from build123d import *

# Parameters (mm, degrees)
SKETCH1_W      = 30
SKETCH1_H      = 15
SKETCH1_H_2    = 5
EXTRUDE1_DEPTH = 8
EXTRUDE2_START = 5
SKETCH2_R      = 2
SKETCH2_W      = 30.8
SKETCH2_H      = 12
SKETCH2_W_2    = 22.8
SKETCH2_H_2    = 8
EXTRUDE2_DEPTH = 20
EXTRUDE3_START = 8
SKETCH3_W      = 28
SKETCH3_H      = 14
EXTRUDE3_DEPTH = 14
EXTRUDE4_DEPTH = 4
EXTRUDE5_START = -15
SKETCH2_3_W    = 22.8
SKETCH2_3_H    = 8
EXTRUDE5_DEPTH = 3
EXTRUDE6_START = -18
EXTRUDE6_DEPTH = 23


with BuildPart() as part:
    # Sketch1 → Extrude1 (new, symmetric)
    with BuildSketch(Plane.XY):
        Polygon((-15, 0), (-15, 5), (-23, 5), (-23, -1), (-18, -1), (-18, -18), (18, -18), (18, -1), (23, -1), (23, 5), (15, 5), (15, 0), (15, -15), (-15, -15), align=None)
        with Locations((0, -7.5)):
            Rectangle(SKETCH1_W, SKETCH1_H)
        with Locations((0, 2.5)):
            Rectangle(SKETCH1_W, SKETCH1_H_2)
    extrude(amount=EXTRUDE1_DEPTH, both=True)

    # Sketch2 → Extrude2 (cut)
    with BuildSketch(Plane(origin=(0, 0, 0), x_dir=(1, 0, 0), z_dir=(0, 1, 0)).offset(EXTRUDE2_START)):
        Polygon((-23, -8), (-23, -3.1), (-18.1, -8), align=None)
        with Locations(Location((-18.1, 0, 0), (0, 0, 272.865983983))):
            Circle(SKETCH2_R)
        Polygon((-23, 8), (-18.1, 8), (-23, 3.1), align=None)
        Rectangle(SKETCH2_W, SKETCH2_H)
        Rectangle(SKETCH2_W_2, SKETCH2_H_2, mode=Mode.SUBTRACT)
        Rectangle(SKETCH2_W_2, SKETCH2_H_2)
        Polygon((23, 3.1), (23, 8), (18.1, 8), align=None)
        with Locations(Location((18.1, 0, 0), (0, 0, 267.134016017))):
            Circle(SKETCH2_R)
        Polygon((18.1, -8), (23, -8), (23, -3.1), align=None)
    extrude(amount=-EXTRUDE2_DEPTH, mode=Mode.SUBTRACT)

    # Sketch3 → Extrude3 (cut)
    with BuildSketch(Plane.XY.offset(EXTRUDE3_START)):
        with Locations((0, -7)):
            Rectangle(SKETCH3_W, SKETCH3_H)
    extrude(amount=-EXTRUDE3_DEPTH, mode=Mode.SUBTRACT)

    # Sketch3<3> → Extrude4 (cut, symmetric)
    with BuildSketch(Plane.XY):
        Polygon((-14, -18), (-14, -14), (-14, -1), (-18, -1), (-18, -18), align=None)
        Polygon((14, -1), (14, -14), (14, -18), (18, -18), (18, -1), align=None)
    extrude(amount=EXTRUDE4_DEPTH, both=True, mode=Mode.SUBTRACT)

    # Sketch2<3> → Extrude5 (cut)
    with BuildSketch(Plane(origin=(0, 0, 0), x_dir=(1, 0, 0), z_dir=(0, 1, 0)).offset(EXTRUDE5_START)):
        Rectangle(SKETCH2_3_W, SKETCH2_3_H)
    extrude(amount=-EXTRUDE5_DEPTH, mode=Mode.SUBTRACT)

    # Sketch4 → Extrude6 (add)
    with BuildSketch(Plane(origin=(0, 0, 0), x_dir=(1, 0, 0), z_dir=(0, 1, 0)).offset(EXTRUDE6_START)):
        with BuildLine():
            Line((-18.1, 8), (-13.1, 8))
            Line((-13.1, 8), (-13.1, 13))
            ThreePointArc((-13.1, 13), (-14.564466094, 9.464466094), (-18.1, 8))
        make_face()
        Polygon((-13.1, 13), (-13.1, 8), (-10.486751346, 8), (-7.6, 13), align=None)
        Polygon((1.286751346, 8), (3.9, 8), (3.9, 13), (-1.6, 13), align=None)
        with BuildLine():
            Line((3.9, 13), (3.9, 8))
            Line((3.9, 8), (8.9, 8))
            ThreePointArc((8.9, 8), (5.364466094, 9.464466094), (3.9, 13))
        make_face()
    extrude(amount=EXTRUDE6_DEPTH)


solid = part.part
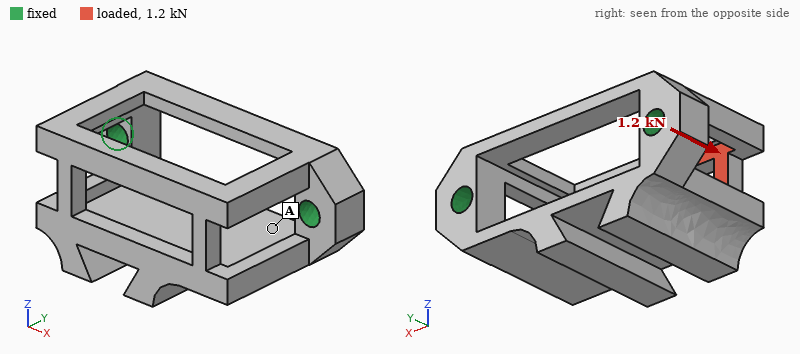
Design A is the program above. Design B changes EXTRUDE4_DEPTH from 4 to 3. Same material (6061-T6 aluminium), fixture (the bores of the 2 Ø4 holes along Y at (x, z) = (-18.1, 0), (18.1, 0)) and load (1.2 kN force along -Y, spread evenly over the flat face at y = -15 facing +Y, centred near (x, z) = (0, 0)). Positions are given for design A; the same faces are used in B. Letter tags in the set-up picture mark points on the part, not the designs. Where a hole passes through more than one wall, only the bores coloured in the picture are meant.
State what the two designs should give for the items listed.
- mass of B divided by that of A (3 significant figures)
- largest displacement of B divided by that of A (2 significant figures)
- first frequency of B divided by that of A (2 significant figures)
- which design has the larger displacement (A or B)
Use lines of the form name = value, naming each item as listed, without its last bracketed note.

mass of B divided by that of A = 1.04
largest displacement of B divided by that of A = 0.91
first frequency of B divided by that of A = 1.1
which design has the larger displacement = A
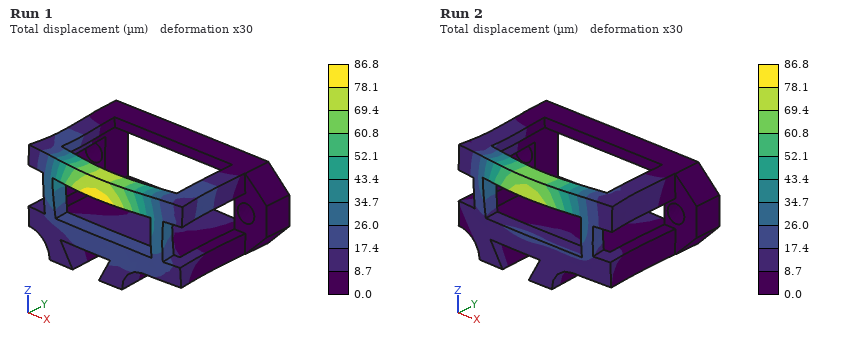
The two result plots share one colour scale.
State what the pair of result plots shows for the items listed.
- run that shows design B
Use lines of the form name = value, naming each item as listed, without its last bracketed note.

run that shows design B = Run 2
